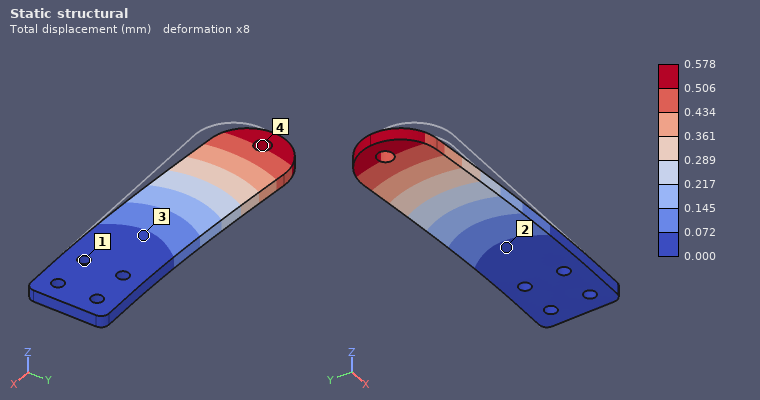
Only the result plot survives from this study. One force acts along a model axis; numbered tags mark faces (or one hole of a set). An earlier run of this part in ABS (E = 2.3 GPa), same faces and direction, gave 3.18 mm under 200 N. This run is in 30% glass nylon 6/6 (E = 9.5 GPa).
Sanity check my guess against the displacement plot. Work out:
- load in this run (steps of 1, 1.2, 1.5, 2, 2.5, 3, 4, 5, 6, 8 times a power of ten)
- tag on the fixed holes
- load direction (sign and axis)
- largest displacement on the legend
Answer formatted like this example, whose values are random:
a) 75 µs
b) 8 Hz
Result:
a) 150 N
b) 1
c) +Y
d) 0.578 mm
